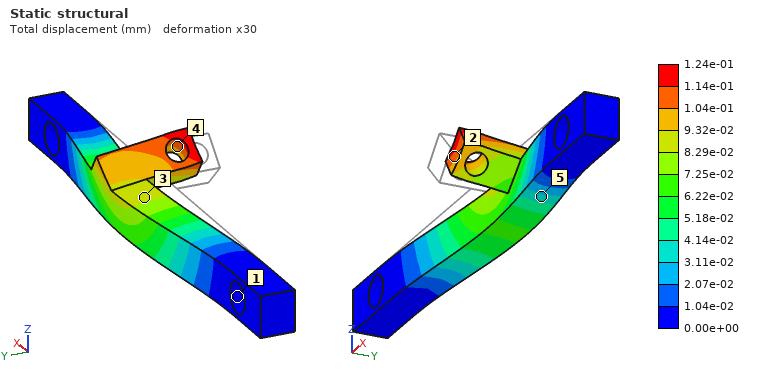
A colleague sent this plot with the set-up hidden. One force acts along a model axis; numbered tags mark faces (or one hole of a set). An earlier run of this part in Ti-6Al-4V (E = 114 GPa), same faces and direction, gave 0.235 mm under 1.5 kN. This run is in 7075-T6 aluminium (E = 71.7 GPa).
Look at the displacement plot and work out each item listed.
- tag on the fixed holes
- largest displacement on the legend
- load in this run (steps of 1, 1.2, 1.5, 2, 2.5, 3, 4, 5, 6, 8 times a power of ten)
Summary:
1
1.24e-01 mm
500 N
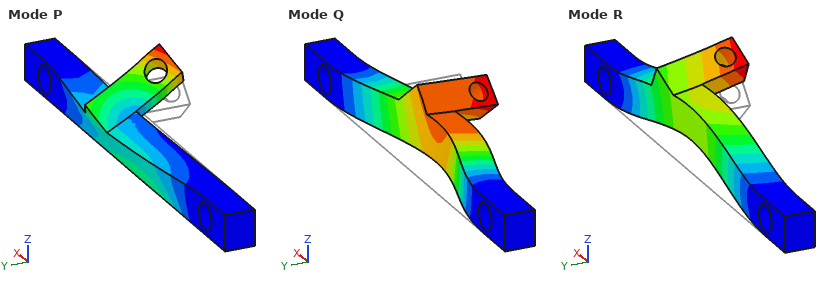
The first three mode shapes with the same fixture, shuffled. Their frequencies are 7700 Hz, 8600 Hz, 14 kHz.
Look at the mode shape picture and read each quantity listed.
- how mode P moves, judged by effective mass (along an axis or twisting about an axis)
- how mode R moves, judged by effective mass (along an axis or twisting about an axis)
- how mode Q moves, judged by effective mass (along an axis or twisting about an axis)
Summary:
twisting about X
along Z
along Y
